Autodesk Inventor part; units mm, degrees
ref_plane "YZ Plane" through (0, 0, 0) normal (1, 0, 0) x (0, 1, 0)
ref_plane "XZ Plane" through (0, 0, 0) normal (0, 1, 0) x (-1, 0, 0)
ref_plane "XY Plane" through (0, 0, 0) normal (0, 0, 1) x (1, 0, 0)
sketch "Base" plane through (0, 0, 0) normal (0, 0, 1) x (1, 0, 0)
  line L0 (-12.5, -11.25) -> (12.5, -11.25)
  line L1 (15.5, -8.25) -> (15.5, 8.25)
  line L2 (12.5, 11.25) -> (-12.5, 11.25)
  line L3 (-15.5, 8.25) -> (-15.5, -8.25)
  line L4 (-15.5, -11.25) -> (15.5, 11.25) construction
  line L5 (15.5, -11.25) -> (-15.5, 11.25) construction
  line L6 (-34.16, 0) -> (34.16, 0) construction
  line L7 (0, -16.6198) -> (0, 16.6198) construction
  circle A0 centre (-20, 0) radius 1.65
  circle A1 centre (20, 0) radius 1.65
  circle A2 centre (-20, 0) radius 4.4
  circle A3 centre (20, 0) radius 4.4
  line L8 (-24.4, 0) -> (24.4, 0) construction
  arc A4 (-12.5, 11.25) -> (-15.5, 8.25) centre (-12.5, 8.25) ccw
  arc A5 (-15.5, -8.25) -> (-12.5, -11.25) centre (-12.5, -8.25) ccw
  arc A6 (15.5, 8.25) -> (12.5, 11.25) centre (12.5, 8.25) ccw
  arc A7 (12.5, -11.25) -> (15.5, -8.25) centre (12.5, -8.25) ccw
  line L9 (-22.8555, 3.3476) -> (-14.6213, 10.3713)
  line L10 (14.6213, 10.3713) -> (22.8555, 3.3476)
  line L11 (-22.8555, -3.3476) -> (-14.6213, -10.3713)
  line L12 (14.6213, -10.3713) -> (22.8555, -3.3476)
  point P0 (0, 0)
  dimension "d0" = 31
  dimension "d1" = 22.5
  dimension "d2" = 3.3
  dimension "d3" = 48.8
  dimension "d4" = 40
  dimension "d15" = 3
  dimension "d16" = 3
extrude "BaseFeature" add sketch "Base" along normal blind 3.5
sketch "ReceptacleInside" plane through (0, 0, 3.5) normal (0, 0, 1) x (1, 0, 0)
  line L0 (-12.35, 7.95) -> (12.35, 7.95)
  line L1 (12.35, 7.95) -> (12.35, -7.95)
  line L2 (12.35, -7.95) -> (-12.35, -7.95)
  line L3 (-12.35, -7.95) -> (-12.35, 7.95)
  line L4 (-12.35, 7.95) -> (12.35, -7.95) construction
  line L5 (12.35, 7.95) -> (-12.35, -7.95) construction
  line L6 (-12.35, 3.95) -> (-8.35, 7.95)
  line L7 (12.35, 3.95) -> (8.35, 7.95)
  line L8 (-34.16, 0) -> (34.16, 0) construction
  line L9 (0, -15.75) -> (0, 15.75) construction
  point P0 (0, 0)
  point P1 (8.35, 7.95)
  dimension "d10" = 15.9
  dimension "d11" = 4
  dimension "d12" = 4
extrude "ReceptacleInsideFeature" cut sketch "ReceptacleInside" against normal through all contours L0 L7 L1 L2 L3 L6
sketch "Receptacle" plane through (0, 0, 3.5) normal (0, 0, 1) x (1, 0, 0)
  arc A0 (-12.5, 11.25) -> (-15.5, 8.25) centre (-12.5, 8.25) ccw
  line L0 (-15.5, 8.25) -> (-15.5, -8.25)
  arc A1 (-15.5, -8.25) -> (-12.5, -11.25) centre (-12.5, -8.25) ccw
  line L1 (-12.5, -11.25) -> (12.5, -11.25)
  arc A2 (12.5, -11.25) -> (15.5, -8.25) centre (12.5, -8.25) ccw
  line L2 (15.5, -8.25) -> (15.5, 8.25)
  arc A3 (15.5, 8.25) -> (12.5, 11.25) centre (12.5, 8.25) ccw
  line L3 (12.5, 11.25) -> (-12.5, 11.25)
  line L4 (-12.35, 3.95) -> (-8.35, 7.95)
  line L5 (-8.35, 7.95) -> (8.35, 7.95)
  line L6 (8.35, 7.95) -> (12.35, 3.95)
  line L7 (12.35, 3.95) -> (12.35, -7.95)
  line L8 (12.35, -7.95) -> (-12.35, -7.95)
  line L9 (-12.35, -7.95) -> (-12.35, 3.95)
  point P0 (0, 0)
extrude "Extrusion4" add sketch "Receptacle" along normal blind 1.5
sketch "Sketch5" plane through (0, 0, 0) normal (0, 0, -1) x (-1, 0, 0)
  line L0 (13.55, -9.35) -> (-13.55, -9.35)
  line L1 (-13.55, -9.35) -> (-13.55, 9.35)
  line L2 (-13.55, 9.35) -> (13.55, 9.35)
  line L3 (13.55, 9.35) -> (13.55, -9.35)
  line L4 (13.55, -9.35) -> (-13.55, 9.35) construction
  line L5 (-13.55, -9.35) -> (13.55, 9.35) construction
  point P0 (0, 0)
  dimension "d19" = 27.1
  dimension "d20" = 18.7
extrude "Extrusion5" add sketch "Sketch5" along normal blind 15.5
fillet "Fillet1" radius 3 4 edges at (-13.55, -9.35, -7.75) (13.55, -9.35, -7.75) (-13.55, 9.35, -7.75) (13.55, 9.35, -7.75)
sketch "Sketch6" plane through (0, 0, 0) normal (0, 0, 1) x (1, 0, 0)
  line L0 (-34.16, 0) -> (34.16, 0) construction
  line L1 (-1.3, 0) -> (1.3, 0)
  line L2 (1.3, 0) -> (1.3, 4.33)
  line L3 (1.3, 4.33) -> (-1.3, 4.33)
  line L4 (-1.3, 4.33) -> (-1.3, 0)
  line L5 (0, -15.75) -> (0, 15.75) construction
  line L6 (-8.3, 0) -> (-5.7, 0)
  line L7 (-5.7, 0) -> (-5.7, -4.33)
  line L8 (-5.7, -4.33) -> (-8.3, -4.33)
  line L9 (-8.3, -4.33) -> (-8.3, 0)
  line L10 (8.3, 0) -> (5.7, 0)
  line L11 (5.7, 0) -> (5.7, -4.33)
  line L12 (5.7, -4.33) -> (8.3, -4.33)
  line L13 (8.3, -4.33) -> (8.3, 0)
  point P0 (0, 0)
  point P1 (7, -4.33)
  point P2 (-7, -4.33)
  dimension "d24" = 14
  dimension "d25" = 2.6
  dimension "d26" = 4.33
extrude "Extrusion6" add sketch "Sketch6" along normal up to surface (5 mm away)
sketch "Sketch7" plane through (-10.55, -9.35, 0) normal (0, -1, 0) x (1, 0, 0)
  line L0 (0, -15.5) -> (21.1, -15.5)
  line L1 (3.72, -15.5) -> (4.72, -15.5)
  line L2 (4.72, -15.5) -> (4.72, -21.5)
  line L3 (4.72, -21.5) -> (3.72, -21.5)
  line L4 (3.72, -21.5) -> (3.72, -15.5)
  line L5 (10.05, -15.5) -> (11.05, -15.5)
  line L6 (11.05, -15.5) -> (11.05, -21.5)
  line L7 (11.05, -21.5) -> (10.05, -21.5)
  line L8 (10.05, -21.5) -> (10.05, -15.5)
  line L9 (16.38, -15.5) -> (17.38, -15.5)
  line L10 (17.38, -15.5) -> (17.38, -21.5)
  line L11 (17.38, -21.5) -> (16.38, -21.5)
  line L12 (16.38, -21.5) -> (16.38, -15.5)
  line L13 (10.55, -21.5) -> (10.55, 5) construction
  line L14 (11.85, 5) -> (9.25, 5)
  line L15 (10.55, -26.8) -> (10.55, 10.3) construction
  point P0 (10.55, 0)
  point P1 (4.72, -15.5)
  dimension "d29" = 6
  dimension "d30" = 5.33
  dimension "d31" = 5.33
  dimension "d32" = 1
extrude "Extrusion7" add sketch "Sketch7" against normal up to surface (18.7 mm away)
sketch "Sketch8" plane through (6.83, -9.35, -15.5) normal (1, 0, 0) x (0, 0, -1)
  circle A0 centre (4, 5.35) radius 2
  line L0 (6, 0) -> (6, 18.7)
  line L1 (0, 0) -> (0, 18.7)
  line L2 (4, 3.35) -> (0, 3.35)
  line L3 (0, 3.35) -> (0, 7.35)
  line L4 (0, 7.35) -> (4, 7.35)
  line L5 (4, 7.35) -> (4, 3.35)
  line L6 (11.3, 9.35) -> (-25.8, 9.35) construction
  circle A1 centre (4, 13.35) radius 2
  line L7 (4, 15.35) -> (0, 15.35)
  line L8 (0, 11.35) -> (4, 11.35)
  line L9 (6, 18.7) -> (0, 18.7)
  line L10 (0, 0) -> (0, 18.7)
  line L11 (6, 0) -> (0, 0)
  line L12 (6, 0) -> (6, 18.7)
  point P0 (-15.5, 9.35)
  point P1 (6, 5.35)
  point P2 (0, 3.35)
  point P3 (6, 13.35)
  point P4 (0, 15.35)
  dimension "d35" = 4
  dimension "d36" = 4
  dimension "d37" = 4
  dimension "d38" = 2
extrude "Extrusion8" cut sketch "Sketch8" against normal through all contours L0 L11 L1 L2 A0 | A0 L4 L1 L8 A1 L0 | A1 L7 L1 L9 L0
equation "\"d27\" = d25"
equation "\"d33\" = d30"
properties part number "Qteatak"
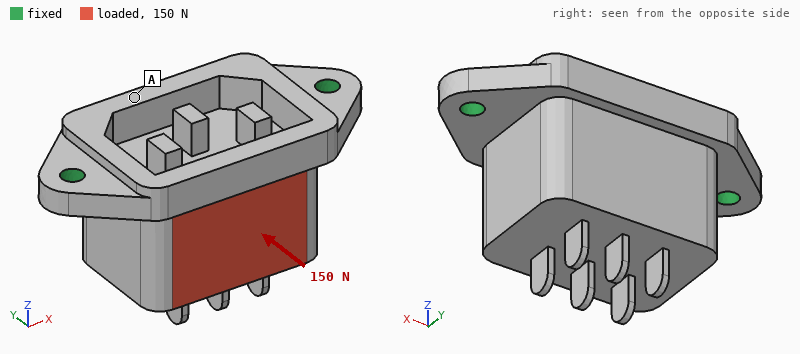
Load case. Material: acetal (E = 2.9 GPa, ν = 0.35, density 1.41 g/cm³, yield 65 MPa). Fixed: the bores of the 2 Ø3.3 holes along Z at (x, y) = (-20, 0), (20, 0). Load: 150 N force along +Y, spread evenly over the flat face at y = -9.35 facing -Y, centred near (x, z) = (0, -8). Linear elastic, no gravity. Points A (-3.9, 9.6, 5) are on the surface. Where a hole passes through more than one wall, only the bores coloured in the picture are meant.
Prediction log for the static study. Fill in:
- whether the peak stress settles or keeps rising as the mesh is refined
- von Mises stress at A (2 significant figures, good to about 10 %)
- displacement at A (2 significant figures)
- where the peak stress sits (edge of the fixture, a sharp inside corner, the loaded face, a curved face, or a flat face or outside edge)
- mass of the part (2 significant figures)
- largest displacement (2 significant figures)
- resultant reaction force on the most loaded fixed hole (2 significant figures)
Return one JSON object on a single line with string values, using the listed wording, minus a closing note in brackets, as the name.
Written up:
{"whether the peak stress settles or keeps rising as the mesh is refined": "keeps rising", "von Mises stress at A": "3.3 MPa", "displacement at A": "0.18 mm", "where the peak stress sits": "edge of the fixture", "mass of the part": "14 g", "largest displacement": "0.45 mm", "resultant reaction force on the most loaded fixed hole": "75 N"}
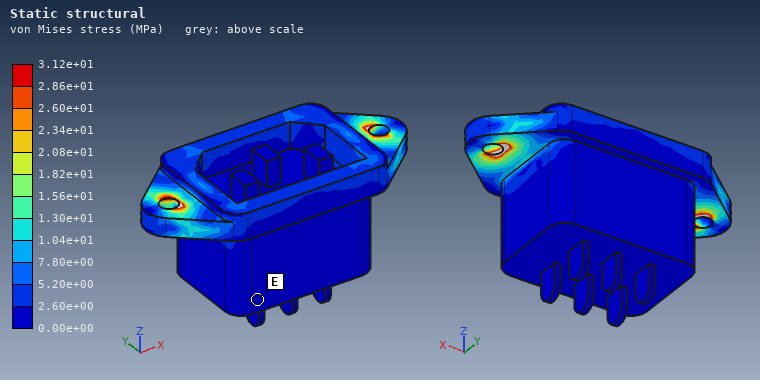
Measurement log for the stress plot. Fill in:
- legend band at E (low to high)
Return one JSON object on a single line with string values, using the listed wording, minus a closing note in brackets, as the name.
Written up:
{"legend band at E": "0.00e+00 to 2.60e+00 MPa"}
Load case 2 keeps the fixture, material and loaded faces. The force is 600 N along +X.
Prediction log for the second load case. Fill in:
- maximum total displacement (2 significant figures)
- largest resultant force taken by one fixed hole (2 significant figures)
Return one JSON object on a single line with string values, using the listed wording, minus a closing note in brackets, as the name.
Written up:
{"maximum total displacement": "0.15 mm", "largest resultant force taken by one fixed hole": "370 N"}
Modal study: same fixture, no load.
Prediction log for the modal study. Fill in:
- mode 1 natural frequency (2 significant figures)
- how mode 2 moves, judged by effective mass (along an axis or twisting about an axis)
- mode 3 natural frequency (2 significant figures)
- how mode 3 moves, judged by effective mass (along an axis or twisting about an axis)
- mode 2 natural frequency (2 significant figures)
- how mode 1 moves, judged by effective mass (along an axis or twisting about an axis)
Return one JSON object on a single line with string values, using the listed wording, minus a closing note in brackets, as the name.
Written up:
{"mode 1 natural frequency": "1000 Hz", "how mode 2 moves, judged by effective mass": "along Z", "mode 3 natural frequency": "3500 Hz", "how mode 3 moves, judged by effective mass": "along X", "mode 2 natural frequency": "2700 Hz", "how mode 1 moves, judged by effective mass": "along Y"}
